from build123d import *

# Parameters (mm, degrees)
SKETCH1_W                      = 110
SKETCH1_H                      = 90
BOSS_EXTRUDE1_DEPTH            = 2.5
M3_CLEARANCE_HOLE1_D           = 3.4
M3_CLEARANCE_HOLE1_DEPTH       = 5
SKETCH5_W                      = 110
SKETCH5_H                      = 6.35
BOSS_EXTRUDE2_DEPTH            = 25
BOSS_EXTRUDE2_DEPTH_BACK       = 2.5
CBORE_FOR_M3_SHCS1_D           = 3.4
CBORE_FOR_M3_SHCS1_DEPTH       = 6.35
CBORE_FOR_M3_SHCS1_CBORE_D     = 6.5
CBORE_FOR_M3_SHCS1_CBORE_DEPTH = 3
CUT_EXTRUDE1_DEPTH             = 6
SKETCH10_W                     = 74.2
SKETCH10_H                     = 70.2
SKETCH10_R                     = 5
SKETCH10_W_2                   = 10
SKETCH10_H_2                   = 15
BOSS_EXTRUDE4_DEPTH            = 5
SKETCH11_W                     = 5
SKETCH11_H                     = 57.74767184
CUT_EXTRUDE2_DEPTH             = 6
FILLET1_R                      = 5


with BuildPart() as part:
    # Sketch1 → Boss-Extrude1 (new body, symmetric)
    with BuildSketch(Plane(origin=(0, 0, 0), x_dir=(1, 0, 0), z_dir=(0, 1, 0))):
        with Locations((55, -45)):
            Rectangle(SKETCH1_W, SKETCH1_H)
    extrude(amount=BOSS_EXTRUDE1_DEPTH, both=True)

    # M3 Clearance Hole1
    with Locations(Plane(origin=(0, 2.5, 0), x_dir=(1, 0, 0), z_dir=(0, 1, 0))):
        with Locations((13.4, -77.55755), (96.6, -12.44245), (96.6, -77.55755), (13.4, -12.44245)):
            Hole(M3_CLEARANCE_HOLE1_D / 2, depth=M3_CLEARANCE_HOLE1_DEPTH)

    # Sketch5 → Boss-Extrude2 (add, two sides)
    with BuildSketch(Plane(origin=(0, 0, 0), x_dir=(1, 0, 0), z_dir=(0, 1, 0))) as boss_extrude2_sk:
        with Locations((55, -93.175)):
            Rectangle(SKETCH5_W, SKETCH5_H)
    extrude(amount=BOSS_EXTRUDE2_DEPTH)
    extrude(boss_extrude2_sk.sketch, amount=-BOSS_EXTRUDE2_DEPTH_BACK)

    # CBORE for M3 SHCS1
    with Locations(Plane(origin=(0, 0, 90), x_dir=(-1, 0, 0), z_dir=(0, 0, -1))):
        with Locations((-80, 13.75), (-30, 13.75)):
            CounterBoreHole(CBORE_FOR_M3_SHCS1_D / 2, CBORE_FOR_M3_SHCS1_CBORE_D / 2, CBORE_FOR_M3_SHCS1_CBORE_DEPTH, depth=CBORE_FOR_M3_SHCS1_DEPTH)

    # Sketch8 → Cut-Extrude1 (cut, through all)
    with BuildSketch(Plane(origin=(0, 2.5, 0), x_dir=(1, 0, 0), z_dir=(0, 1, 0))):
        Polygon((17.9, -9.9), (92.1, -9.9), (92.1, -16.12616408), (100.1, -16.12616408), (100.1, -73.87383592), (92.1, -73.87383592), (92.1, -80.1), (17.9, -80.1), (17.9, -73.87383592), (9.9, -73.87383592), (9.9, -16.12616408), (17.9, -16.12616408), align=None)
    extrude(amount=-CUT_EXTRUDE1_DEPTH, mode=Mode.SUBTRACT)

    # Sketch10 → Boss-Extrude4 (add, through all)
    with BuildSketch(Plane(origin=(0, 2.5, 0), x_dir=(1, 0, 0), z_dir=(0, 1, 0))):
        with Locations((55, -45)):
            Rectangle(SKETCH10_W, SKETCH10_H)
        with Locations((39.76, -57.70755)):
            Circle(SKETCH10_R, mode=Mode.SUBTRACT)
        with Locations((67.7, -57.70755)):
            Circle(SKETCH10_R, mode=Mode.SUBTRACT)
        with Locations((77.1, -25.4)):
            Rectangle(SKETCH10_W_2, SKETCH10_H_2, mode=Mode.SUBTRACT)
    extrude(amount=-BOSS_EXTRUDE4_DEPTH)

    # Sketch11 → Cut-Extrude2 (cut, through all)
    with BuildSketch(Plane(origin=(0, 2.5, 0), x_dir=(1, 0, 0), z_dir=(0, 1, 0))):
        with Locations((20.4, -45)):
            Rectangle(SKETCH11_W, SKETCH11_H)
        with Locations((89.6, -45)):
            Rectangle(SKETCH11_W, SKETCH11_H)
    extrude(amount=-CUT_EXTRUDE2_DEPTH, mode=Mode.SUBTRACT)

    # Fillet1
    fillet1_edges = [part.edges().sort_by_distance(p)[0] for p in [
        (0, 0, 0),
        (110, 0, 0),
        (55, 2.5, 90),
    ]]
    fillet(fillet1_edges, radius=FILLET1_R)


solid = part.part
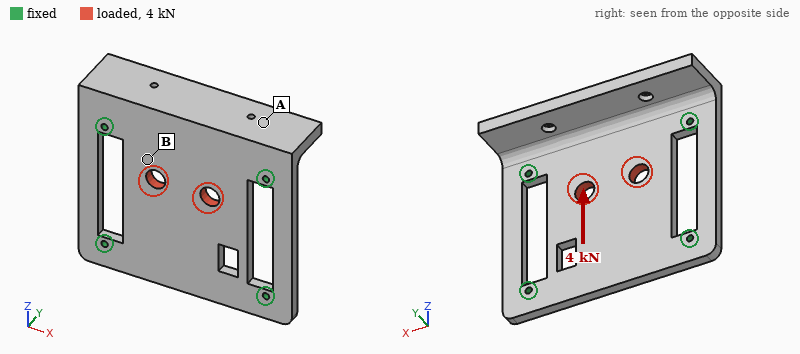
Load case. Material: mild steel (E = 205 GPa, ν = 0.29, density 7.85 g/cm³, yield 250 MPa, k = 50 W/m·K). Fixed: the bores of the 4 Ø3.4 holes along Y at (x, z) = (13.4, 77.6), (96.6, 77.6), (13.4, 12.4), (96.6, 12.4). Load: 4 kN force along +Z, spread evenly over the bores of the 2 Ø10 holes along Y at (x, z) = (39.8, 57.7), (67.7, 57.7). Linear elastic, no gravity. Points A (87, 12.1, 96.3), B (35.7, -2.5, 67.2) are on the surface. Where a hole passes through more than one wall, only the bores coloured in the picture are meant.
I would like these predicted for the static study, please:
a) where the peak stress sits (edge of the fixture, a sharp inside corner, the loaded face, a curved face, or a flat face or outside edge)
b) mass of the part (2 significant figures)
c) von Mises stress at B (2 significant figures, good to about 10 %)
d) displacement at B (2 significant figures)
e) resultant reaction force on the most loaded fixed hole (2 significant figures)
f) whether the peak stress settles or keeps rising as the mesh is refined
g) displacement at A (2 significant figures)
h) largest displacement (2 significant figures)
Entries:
edge of the fixture
470 g
14 MPa
6.1 µm
1.3 kN
keeps rising
3.9 µm
8.0 µm
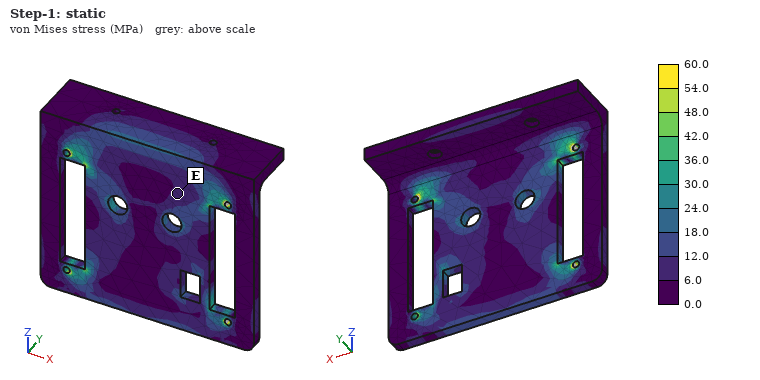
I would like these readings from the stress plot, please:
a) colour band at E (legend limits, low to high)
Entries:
6.0 to 12.0 MPa
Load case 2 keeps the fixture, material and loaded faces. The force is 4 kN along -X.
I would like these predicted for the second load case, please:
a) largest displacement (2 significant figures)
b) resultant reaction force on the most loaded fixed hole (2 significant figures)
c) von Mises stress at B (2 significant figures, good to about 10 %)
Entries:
5.4 µm
1.4 kN
22 MPa
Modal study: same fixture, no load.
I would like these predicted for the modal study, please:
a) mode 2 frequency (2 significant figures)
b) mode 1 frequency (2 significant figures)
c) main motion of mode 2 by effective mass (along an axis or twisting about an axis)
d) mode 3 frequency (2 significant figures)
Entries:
2900 Hz
2200 Hz
along Y
4000 Hz
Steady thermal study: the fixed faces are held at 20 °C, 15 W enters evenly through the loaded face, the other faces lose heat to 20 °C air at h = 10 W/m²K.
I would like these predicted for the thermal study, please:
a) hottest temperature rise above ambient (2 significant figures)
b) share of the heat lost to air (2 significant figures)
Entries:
28 K
19 %
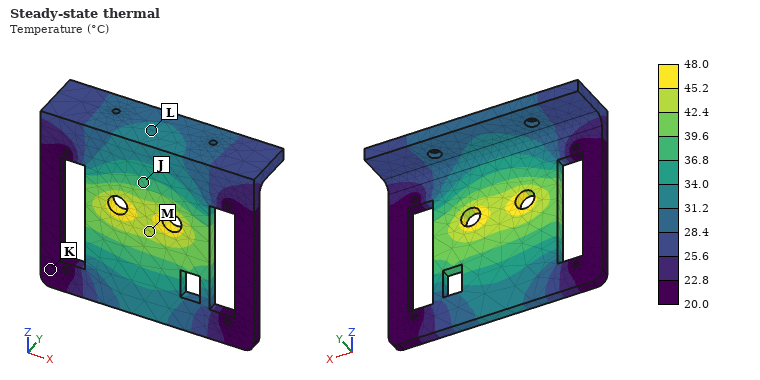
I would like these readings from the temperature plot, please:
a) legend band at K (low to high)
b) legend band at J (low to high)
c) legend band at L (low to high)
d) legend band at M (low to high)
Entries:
20.0 to 22.8 °C
36.8 to 39.6 °C
31.2 to 34.0 °C
42.4 to 45.2 °C
